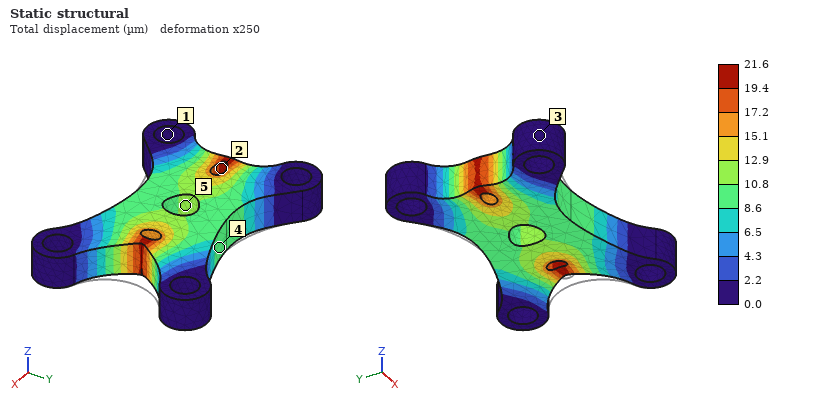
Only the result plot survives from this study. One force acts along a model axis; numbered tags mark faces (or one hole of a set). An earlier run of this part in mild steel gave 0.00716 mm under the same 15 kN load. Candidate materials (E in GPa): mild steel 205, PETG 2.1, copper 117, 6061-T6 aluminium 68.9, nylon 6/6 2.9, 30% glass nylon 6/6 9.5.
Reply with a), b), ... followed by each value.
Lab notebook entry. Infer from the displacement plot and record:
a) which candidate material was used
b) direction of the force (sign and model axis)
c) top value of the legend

a) 6061-T6 aluminium
b) -X
c) 21.6 µm
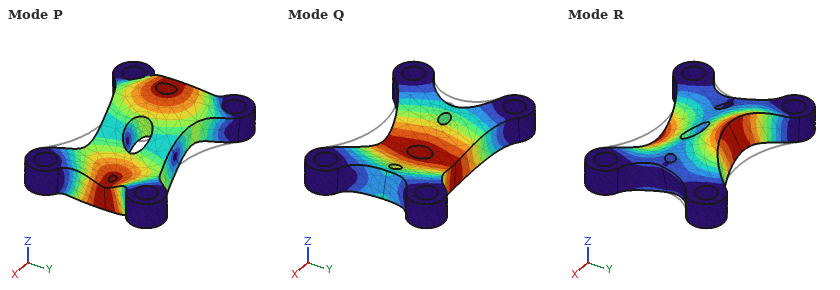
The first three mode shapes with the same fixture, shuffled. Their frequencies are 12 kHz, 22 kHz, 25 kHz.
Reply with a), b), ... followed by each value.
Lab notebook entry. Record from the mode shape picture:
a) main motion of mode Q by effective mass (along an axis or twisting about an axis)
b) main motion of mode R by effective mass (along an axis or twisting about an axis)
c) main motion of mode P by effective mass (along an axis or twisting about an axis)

a) along Z
b) twisting about X
c) twisting about Y
